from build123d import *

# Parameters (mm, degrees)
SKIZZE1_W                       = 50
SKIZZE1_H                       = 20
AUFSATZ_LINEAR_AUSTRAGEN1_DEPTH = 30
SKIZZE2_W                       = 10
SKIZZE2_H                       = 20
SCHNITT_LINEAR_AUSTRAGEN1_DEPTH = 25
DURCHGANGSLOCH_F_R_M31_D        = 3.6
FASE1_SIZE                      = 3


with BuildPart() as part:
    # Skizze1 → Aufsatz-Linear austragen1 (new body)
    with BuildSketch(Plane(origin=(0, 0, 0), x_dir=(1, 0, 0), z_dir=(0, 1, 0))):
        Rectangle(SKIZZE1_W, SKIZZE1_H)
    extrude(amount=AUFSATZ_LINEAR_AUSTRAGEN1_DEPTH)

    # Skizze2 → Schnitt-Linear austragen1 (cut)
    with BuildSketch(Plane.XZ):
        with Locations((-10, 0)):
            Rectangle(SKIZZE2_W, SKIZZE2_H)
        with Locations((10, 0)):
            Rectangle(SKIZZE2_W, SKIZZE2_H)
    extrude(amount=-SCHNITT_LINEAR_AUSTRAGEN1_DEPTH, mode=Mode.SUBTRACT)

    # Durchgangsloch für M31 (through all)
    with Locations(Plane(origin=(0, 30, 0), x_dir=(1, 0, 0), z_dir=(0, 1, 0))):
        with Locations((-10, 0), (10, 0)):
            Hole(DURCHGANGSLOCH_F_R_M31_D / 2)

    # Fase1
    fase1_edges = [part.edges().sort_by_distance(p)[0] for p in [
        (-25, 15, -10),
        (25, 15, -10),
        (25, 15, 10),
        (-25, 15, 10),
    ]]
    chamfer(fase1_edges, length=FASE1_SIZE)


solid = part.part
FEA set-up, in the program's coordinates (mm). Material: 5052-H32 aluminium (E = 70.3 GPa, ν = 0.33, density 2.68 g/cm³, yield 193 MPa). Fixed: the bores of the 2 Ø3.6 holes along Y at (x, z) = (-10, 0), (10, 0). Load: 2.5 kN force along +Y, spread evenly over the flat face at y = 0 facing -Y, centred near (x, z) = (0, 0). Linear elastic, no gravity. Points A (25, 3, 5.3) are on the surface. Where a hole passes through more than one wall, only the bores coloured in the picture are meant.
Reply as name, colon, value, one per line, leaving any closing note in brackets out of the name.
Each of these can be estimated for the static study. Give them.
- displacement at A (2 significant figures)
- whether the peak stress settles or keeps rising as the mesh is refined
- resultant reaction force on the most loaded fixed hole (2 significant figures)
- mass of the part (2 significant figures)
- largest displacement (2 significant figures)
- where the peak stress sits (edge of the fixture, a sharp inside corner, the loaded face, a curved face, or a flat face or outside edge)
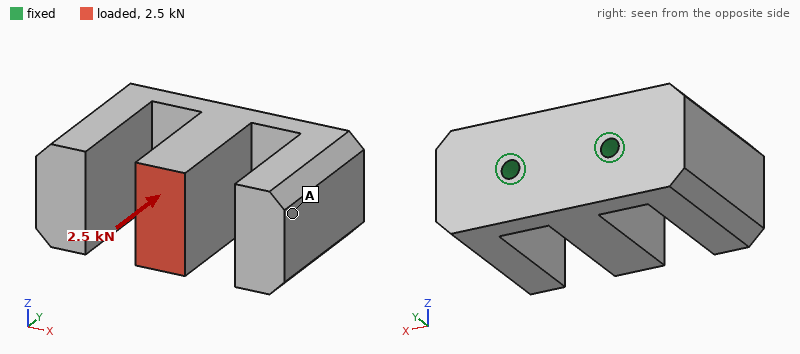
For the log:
displacement at A: 13 µm
whether the peak stress settles or keeps rising as the mesh is refined: keeps rising
resultant reaction force on the most loaded fixed hole: 1.3 kN
mass of the part: 52 g
largest displacement: 14 µm
where the peak stress sits: edge of the fixture
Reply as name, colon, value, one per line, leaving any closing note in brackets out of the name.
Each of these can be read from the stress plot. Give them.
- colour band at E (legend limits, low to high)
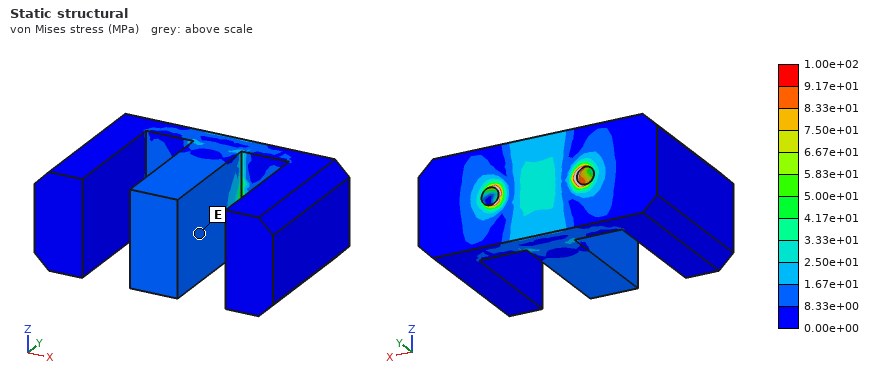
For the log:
colour band at E: 8.33e+00 to 1.67e+01 MPa
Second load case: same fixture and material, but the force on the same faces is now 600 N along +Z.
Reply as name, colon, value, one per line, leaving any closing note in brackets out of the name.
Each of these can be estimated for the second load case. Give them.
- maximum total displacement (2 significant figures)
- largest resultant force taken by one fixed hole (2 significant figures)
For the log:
maximum total displacement: 82 µm
largest resultant force taken by one fixed hole: 300 N
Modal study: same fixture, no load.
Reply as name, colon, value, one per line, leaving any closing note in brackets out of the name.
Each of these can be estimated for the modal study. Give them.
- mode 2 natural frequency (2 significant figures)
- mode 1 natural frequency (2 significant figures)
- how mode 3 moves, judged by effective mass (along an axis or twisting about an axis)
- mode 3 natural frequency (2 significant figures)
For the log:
mode 2 natural frequency: 3300 Hz
mode 1 natural frequency: 3200 Hz
how mode 3 moves, judged by effective mass: along Z
mode 3 natural frequency: 4100 Hz
